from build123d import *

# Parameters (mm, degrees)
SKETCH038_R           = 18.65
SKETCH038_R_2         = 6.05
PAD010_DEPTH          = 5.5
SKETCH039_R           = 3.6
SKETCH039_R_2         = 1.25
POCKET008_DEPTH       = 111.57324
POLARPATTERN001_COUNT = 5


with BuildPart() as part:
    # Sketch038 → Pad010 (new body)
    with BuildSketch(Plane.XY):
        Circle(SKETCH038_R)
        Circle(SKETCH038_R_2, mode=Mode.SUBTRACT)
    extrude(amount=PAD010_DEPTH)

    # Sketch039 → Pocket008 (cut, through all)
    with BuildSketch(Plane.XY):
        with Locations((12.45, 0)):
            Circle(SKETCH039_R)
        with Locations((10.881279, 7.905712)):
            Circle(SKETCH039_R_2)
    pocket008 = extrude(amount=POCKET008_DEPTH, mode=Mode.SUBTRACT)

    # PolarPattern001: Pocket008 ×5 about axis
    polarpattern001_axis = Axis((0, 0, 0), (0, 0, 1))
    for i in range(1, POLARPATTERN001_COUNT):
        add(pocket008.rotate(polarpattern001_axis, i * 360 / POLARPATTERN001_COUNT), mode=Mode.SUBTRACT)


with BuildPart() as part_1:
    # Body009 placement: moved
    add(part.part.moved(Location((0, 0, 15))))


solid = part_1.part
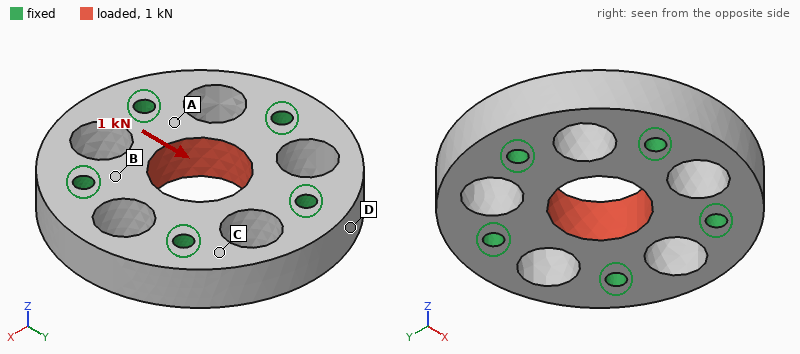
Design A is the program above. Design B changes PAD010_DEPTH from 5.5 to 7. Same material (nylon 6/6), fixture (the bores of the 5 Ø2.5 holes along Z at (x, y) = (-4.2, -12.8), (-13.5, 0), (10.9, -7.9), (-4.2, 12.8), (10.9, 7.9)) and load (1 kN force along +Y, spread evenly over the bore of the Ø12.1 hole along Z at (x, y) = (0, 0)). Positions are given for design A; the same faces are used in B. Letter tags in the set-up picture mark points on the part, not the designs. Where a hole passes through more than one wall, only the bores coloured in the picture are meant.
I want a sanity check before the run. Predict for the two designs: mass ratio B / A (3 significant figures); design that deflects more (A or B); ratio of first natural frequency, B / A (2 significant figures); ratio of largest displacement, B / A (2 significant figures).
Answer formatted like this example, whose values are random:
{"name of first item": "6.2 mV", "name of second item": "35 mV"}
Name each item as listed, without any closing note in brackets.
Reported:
{"mass ratio B / A": "1.27", "design that deflects more": "A", "ratio of first natural frequency, B / A": "1.1", "ratio of largest displacement, B / A": "0.78"}
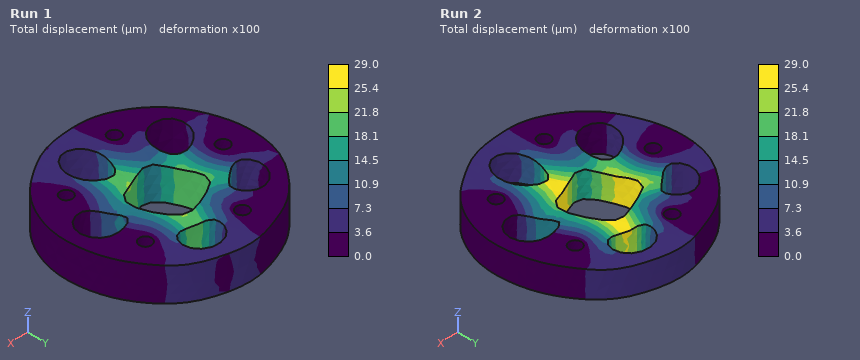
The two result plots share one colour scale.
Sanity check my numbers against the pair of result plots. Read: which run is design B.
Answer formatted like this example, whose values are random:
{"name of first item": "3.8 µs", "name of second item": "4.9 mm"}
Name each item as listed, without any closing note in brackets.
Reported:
{"which run is design B": "Run 1"}
